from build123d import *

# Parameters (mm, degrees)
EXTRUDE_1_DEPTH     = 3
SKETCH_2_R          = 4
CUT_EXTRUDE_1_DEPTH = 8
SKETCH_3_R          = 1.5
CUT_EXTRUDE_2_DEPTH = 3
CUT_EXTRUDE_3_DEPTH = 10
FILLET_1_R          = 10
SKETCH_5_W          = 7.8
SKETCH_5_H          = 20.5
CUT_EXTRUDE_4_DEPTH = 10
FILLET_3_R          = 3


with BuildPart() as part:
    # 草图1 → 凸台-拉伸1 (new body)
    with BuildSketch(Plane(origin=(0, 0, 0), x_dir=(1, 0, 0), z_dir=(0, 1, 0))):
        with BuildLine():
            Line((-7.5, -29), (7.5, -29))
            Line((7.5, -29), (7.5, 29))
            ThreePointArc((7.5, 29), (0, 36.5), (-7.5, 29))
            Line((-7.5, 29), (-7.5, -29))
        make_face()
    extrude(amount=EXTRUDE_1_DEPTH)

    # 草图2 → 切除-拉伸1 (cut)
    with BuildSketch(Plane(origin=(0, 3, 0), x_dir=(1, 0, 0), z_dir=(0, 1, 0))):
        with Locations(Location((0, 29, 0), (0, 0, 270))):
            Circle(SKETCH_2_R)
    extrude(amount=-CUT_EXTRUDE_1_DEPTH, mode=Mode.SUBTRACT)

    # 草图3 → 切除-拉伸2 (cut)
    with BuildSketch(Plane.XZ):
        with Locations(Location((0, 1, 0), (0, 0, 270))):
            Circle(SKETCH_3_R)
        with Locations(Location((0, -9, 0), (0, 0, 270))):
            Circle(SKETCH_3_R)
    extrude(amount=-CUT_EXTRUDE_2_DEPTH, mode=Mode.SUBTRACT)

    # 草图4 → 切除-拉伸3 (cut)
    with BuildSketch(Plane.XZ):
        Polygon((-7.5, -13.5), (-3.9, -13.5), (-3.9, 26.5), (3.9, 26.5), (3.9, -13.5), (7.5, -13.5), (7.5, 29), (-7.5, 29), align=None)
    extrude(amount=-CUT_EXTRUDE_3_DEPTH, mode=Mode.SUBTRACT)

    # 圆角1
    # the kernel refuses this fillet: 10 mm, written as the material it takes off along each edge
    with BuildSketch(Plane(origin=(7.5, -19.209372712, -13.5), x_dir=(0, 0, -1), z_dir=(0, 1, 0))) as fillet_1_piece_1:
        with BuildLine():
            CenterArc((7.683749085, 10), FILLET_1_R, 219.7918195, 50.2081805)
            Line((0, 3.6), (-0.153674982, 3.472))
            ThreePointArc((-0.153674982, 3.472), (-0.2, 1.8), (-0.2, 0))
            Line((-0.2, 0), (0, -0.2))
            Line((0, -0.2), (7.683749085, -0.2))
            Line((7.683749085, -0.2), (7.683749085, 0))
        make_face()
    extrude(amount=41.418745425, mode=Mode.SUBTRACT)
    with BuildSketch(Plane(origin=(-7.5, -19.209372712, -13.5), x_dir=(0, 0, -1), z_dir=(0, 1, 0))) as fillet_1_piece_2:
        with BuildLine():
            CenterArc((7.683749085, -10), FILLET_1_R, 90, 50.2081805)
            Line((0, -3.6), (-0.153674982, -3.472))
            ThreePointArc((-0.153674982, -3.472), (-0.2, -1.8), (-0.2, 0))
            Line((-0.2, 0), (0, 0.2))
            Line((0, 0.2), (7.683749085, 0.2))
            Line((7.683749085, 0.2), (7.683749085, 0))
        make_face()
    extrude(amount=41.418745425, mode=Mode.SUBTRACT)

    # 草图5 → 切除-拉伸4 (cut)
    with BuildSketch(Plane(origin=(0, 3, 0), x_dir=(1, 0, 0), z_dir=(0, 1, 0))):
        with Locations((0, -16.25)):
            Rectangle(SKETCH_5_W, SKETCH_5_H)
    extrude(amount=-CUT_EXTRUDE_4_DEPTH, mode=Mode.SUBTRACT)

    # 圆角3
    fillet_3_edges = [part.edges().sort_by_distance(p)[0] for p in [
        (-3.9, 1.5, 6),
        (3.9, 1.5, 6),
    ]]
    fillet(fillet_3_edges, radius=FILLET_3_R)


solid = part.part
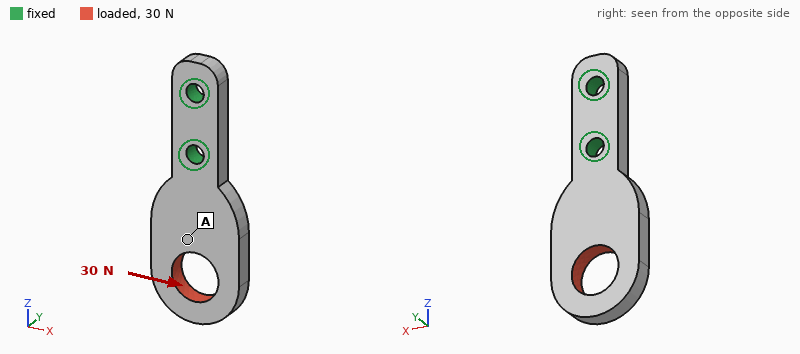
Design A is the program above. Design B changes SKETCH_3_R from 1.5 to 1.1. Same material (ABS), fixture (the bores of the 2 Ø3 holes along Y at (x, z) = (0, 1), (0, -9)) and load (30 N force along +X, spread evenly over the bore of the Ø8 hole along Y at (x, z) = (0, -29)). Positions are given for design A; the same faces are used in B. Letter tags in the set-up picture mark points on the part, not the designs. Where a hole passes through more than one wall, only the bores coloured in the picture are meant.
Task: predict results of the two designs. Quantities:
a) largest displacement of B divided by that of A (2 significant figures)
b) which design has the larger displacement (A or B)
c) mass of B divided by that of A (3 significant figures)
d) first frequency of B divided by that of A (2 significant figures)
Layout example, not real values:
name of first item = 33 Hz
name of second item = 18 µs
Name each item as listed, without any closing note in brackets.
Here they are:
largest displacement of B divided by that of A = 1.1
which design has the larger displacement = B
mass of B divided by that of A = 1.02
first frequency of B divided by that of A = 0.95
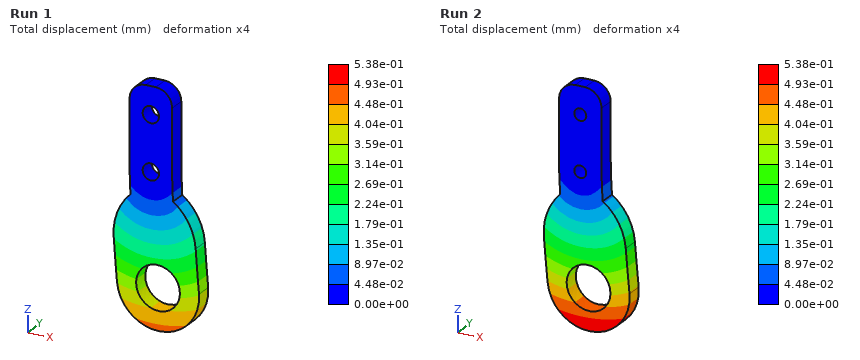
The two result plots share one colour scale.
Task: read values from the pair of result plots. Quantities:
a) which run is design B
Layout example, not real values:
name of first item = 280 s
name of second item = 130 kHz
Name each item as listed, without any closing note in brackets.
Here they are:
which run is design B = Run 2
